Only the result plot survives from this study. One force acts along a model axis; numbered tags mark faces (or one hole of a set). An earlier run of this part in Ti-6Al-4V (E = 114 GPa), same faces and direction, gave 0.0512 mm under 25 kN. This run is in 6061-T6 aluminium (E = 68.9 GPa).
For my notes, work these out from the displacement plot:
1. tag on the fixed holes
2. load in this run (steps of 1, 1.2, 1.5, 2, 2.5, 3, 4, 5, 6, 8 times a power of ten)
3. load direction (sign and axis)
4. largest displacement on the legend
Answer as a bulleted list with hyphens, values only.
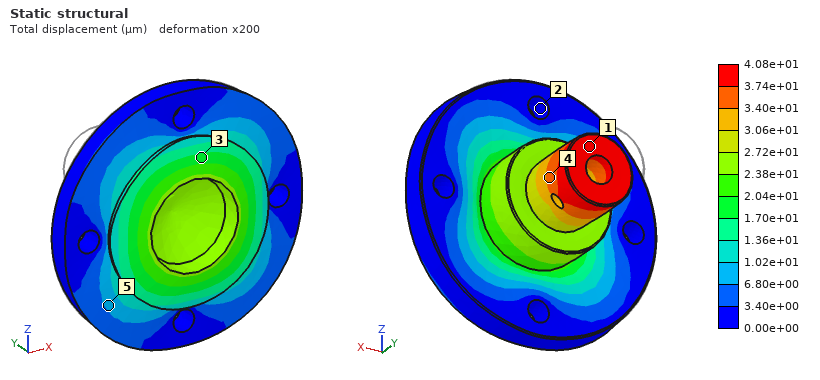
- 2
- 12 kN
- -Y
- 4.08e+01 µm
